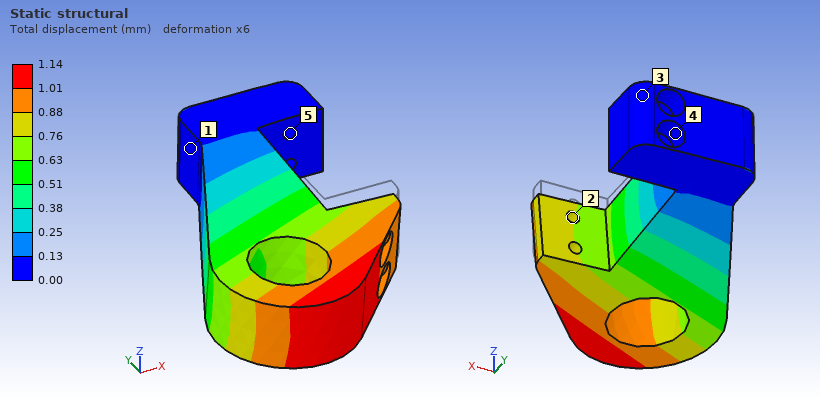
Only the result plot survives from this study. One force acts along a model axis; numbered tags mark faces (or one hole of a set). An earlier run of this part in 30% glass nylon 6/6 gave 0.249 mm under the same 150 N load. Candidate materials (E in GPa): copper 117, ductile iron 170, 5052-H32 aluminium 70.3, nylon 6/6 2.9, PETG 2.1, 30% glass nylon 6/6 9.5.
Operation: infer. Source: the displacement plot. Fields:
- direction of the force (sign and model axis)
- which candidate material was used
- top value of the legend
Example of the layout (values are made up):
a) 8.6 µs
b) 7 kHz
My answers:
a) -Z
b) PETG
c) 1.14 mm
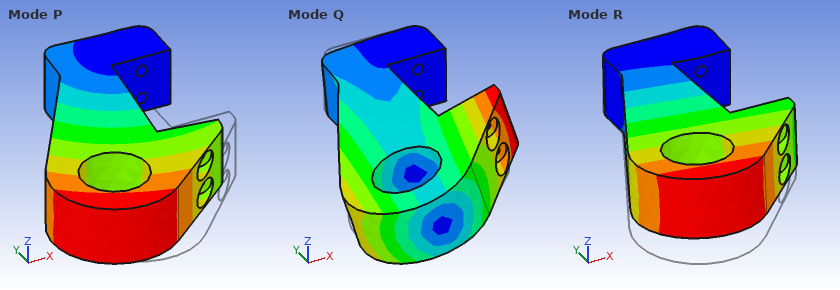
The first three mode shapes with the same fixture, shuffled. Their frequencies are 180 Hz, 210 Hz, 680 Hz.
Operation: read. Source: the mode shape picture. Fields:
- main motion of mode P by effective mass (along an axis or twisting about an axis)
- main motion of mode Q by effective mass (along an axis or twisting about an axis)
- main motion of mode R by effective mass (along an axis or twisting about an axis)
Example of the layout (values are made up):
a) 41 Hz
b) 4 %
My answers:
a) along X
b) twisting about Y
c) along Z
